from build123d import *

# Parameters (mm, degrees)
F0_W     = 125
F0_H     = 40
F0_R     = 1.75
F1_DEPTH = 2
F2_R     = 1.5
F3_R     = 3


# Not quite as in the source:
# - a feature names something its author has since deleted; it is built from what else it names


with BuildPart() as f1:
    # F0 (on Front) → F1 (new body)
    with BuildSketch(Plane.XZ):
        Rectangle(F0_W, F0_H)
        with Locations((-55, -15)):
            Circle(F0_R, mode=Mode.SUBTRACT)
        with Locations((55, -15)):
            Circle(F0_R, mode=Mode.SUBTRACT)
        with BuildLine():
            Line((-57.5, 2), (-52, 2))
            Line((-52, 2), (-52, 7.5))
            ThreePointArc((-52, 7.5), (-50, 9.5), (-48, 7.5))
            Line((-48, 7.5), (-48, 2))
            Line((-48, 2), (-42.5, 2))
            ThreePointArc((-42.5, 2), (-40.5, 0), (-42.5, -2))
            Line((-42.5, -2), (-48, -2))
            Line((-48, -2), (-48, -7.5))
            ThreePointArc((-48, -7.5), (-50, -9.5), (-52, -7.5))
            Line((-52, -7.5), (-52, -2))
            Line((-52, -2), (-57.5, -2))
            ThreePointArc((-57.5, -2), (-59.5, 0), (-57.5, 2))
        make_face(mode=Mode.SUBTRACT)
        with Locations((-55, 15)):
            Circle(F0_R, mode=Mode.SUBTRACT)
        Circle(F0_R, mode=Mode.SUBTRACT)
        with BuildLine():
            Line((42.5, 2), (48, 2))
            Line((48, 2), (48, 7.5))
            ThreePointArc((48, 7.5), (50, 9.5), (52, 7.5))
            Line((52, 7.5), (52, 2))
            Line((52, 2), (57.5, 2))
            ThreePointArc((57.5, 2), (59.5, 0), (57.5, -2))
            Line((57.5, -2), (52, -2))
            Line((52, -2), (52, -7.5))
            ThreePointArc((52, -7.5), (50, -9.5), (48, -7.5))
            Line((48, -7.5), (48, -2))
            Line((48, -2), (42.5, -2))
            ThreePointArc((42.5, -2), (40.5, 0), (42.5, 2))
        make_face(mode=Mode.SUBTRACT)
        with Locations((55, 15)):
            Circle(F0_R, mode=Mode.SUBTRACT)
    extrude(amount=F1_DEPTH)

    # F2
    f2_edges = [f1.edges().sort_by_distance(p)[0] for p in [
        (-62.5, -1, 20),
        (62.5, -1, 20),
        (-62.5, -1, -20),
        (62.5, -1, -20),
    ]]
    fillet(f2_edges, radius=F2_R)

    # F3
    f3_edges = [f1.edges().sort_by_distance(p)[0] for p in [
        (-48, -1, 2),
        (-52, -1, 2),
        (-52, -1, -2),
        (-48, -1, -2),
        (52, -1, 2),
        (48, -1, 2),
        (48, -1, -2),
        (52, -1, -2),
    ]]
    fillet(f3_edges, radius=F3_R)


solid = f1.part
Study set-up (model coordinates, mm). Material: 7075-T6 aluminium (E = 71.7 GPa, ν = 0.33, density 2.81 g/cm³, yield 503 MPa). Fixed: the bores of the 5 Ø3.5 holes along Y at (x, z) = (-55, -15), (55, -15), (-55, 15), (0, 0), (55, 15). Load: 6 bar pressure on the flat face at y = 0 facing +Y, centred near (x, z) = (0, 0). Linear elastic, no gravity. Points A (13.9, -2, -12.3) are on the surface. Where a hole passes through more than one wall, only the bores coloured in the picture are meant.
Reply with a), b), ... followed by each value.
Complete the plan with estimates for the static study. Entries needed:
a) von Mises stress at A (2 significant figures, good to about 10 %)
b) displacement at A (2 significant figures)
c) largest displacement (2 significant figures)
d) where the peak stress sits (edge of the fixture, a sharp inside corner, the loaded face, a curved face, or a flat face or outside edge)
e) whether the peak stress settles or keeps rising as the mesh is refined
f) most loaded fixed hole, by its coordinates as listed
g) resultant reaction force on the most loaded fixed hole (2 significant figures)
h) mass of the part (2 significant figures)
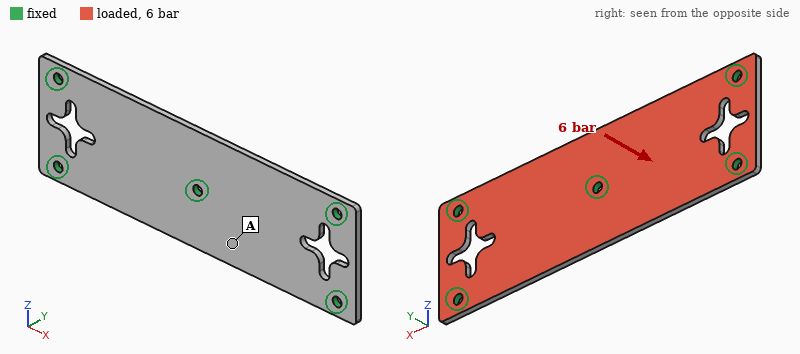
a) 58 MPa
b) 0.27 mm
c) 0.41 mm
d) edge of the fixture
e) keeps rising
f) (0, 0)
g) 1.4 kN
h) 26 g
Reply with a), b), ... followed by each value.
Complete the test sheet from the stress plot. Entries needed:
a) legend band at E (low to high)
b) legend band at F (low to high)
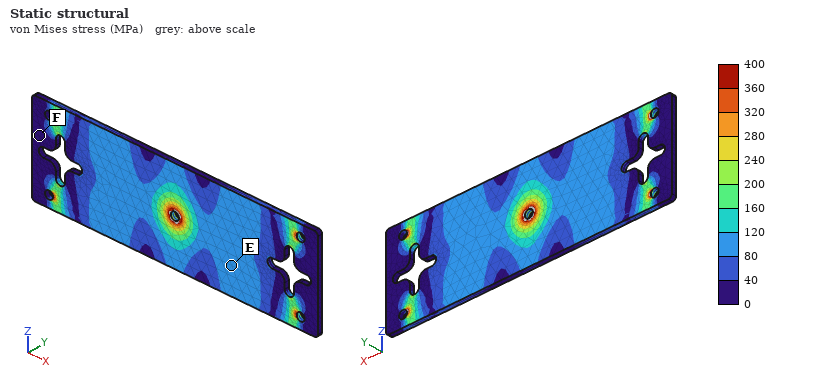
a) 80 to 120 MPa
b) 0 to 40 MPa
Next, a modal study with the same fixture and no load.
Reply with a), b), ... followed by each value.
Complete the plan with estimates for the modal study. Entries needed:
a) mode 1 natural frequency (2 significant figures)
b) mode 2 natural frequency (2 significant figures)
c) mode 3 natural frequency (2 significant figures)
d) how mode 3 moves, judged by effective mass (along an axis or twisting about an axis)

a) 2800 Hz
b) 2900 Hz
c) 3100 Hz
d) along Y
